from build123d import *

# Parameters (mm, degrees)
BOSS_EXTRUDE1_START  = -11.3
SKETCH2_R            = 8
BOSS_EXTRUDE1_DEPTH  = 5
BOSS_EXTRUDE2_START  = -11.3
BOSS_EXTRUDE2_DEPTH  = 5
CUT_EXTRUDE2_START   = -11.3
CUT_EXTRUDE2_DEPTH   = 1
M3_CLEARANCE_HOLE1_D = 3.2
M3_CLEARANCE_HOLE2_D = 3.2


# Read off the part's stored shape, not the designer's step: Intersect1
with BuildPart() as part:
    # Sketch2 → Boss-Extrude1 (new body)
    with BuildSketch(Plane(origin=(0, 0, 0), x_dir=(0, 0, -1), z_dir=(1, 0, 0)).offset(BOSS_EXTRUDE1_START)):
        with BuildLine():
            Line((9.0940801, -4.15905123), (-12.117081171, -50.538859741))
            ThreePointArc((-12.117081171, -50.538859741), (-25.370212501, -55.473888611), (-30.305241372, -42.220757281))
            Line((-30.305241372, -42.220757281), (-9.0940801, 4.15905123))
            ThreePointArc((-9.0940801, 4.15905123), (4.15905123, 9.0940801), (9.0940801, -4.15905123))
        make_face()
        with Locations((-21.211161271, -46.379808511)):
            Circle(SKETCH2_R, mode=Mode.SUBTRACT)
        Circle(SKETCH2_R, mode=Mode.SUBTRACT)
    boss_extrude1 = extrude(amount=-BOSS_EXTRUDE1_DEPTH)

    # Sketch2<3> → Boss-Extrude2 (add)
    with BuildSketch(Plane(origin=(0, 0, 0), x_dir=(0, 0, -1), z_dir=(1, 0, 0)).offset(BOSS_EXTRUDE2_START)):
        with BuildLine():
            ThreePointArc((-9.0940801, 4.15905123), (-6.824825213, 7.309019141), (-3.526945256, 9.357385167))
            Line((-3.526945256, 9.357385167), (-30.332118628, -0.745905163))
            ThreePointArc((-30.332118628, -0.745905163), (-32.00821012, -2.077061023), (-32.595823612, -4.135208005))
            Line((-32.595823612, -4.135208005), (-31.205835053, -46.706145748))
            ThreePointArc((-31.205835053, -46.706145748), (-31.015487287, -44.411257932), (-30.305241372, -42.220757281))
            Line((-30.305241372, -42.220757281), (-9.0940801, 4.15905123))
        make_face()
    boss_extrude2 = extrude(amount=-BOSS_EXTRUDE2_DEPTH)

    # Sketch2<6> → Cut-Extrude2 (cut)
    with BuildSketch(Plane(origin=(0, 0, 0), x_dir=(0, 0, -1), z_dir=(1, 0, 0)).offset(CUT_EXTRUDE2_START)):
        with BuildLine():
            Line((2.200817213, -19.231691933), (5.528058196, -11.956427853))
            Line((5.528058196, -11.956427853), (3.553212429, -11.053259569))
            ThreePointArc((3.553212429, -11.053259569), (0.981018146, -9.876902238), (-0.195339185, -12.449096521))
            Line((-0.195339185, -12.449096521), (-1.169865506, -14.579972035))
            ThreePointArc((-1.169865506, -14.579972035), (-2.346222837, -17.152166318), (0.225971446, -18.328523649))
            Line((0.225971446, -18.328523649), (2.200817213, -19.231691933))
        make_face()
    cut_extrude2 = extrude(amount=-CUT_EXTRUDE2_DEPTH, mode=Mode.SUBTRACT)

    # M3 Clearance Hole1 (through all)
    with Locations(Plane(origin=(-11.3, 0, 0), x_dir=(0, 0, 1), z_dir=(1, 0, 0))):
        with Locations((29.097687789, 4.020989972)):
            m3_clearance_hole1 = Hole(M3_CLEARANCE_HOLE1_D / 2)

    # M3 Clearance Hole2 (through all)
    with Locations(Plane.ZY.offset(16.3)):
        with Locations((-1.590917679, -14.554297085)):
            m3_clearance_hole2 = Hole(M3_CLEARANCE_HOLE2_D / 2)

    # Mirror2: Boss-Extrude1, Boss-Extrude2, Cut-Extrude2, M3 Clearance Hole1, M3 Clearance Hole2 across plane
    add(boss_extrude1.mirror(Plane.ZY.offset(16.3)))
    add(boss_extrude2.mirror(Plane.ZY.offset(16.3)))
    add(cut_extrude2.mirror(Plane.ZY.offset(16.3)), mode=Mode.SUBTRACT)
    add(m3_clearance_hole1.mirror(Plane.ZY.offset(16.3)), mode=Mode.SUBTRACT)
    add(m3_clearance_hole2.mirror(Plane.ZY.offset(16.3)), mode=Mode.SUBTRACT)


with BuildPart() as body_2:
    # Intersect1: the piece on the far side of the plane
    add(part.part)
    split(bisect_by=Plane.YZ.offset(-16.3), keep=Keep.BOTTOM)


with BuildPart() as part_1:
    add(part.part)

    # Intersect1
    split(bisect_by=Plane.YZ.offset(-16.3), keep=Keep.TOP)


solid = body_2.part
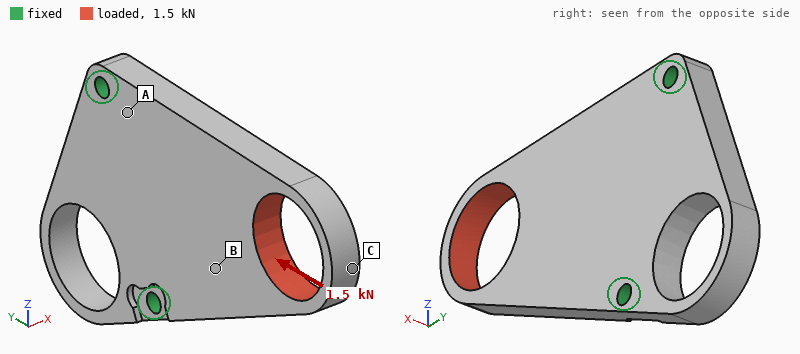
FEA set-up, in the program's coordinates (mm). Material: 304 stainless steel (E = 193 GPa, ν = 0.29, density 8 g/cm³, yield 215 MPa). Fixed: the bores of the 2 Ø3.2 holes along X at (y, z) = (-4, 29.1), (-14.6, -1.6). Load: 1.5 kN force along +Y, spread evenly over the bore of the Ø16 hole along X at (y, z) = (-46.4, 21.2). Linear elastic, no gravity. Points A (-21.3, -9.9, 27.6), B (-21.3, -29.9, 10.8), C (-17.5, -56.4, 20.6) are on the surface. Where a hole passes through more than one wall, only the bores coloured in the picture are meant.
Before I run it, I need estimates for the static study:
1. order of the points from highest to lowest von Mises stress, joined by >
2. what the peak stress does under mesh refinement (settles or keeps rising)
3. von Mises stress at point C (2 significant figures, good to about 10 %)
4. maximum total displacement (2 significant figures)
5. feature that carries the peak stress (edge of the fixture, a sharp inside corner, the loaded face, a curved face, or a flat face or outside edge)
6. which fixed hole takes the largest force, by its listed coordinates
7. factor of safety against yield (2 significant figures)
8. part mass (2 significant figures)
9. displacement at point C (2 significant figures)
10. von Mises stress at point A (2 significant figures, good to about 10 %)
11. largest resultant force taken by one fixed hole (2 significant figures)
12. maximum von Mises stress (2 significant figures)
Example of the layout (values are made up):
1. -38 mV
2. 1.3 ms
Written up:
1. C > A > B
2. settles
3. 73 MPa
4. 17 µm
5. the loaded face
6. (-4, 29.1)
7. 1.8
8. 58 g
9. 17 µm
10. 25 MPa
11. 1.1 kN
12. 120 MPa
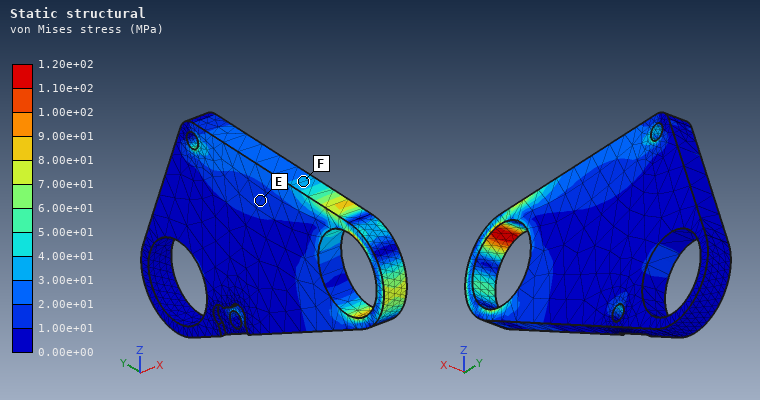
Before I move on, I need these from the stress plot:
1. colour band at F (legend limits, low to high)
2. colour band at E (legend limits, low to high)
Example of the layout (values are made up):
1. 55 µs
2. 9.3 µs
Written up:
1. 3.00e+01 to 4.00e+01 MPa
2. 1.00e+01 to 2.00e+01 MPa
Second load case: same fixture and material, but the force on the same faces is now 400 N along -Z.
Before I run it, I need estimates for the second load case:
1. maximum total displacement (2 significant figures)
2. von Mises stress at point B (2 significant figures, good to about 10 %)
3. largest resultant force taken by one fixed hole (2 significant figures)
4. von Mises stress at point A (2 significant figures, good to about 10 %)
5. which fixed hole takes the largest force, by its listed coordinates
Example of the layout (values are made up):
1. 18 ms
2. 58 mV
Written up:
1. 17 µm
2. 5.0 MPa
3. 550 N
4. 8.5 MPa
5. (-14.6, -1.6)
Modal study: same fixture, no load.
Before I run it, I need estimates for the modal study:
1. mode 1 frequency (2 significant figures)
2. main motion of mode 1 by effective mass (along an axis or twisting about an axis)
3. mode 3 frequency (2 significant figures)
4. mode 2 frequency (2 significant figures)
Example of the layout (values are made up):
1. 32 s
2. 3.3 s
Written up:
1. 2600 Hz
2. along X
3. 9100 Hz
4. 8300 Hz
